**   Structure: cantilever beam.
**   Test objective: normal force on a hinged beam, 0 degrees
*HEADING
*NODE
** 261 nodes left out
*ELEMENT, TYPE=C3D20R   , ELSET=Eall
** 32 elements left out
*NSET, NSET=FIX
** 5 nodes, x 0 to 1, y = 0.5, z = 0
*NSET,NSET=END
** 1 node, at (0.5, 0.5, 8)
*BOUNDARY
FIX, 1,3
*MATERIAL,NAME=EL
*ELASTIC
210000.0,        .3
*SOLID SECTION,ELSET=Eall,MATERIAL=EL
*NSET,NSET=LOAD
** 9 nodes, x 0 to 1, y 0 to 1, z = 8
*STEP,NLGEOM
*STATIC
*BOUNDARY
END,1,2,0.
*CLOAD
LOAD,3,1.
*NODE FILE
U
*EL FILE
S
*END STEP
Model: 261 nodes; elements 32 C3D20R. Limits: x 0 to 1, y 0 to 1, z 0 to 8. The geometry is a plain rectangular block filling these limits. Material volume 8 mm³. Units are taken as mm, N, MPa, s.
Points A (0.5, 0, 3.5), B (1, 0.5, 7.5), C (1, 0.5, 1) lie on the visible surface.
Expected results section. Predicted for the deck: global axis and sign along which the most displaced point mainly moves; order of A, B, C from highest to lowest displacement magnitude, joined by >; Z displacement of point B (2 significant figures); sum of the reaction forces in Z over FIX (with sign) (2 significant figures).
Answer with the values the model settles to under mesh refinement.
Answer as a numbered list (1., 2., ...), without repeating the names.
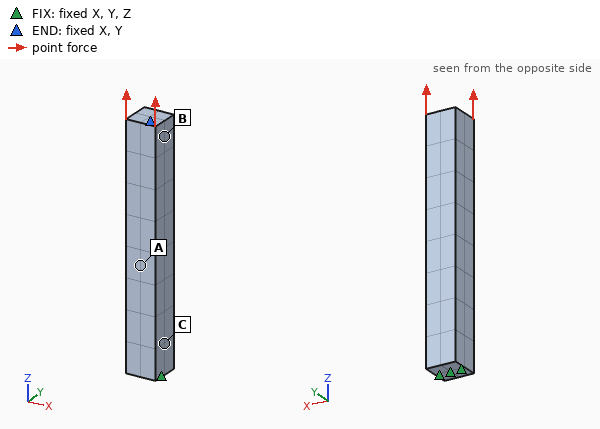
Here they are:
1. +Z
2. B > A > C
3. 3.7e-04 mm
4. -9.0 N
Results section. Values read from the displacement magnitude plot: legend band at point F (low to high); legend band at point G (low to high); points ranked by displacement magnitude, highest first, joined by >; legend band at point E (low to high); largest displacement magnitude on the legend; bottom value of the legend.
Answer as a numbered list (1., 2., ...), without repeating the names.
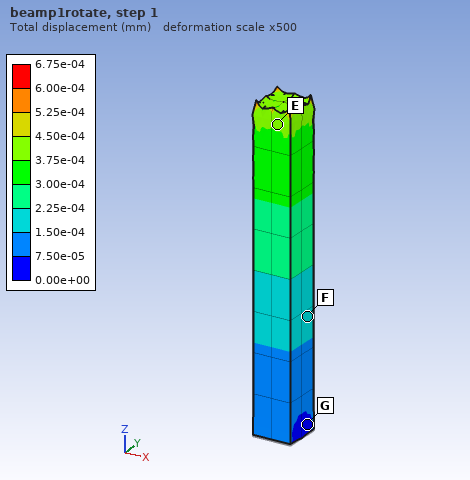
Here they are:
1. 1.50e-04 to 2.25e-04 mm
2. 0.00e+00 to 7.50e-05 mm
3. E > F > G
4. 3.75e-04 to 4.50e-04 mm
5. 6.75e-04 mm
6. 0.00e+00 mm
